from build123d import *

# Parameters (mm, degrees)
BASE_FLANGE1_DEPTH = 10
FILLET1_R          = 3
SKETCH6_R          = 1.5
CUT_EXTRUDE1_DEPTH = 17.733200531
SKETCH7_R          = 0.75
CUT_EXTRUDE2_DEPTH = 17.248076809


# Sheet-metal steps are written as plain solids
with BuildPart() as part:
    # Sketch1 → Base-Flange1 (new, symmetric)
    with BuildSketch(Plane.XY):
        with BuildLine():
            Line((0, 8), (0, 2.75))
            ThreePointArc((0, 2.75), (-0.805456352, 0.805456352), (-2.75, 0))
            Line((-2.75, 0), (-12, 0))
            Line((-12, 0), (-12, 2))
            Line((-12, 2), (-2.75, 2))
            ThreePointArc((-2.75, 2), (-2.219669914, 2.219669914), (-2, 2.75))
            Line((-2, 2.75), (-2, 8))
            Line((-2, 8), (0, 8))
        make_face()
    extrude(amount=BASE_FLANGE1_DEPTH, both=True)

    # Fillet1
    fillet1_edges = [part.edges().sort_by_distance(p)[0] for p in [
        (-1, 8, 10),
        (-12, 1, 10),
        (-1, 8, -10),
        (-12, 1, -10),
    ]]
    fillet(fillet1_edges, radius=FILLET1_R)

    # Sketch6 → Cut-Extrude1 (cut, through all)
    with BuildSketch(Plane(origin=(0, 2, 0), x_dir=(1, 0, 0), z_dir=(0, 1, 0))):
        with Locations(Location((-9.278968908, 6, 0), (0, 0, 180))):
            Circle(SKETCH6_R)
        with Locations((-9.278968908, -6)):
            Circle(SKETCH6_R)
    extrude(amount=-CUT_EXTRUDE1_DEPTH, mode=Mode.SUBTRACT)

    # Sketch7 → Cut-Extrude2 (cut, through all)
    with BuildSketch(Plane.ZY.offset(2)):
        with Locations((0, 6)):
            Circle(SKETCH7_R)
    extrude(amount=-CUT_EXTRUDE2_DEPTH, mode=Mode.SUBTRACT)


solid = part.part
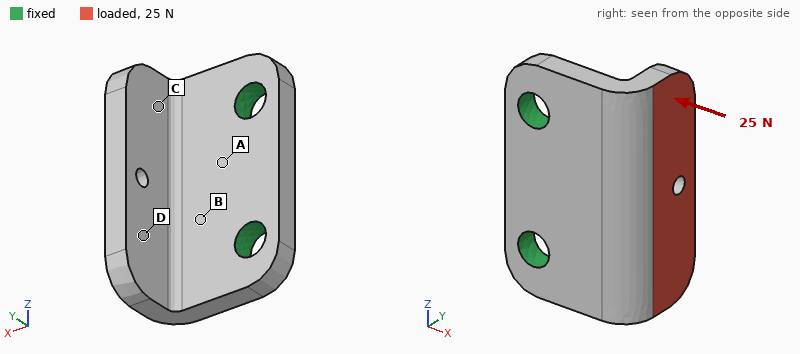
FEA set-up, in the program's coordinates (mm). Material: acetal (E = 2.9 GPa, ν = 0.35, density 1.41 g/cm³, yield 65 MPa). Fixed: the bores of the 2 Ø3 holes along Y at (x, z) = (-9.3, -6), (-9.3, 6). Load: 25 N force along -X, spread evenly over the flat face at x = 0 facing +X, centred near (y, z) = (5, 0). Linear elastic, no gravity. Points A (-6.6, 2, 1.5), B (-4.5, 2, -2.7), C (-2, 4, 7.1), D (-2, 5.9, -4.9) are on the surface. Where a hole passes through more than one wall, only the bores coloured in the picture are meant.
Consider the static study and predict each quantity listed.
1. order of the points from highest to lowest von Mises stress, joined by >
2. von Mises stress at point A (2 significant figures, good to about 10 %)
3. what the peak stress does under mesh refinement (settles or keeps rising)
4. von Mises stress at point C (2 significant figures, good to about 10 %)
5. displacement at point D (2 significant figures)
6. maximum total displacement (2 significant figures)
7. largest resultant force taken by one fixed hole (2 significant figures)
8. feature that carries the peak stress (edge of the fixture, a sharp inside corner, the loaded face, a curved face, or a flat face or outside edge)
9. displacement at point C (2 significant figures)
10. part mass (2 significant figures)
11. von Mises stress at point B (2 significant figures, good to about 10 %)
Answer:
B > A > C > D
5.9 MPa
keeps rising
2.4 MPa
0.12 mm
0.19 mm
13 N
edge of the fixture
0.083 mm
0.91 g
7.5 MPa
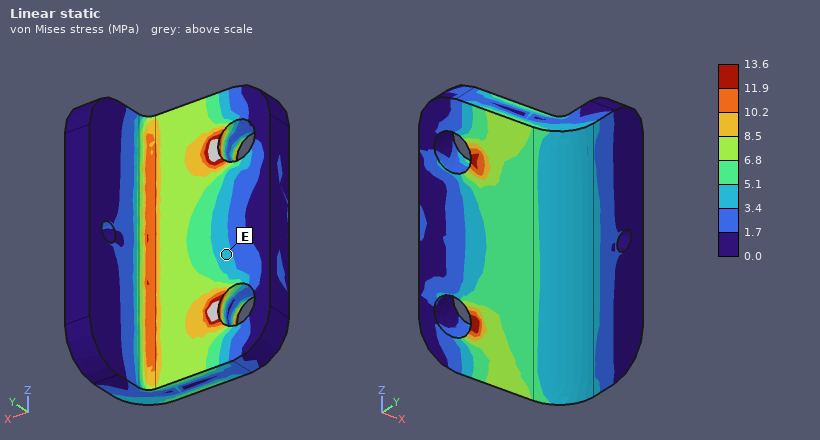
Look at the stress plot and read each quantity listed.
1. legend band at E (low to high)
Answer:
3.4 to 5.1 MPa
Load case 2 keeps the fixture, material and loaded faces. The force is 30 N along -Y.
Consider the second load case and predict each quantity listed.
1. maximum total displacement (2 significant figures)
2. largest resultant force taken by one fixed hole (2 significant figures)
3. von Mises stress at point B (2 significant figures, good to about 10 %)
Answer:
0.26 mm
15 N
8.7 MPa
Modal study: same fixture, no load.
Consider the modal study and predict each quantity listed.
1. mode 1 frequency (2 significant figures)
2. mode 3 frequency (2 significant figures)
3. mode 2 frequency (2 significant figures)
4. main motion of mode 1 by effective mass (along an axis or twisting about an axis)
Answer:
3100 Hz
8800 Hz
4900 Hz
along Y
